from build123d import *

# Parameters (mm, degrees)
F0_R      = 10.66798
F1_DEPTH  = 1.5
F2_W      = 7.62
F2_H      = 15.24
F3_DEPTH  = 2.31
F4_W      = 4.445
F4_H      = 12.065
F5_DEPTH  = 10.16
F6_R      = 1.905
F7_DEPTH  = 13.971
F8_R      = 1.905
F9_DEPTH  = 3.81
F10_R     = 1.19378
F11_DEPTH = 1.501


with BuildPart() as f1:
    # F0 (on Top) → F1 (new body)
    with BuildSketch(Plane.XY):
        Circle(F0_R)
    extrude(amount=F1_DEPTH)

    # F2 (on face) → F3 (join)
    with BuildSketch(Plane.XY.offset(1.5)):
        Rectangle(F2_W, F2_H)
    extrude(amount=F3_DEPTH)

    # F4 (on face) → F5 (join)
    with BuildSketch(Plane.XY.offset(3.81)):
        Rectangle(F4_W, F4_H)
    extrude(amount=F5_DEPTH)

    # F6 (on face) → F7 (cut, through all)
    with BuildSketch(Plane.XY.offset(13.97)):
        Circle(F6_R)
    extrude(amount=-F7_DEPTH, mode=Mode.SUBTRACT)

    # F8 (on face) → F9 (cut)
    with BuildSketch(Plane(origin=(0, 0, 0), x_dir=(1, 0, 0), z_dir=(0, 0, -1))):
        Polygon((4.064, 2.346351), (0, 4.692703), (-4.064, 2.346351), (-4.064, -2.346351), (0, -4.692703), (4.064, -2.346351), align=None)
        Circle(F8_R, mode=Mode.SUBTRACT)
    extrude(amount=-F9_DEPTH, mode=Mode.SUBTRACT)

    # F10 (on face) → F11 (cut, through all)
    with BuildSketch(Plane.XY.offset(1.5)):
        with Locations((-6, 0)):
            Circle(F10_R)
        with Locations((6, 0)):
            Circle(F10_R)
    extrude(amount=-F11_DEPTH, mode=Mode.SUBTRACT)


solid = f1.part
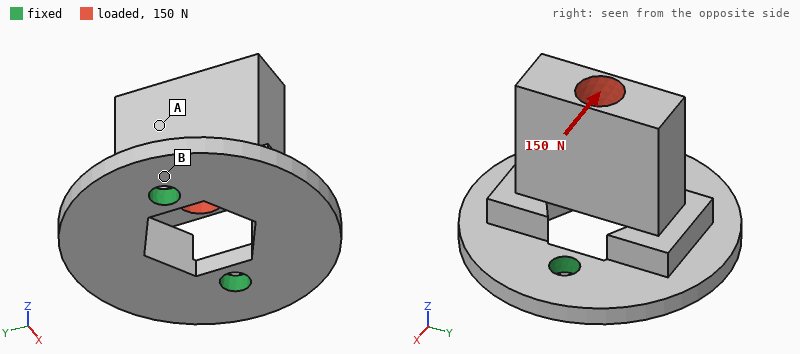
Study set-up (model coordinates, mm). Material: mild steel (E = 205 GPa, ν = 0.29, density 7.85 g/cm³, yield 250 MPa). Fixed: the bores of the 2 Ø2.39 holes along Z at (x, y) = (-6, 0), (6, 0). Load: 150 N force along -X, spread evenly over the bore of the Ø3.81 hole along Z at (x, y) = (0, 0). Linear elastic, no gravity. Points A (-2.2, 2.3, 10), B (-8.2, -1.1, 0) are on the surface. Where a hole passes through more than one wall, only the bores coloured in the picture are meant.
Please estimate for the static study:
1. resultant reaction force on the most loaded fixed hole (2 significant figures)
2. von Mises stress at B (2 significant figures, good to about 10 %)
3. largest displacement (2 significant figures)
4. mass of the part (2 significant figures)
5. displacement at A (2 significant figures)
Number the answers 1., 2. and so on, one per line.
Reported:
1. 130 N
2. 23 MPa
3. 10 µm
4. 7.9 g
5. 6.8 µm
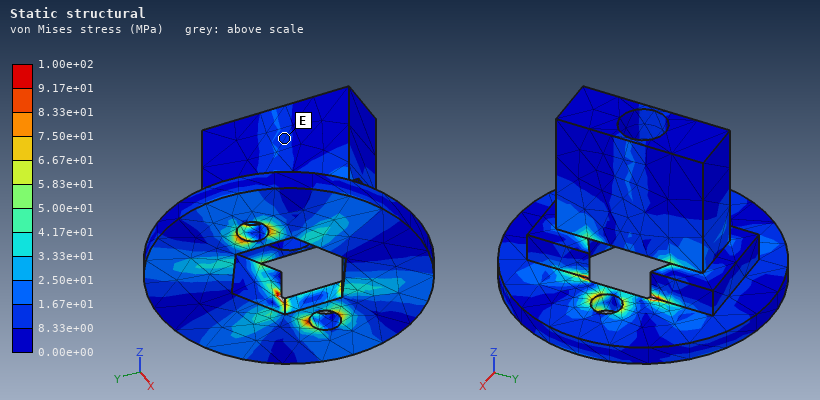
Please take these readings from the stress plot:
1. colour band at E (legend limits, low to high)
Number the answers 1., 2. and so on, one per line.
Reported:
1. 8.33e+00 to 1.67e+01 MPa
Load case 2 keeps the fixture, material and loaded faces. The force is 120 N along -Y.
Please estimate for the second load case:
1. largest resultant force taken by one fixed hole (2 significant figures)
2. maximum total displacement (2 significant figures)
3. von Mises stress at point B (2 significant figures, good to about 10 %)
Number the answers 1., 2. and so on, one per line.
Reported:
1. 60 N
2. 18 µm
3. 29 MPa
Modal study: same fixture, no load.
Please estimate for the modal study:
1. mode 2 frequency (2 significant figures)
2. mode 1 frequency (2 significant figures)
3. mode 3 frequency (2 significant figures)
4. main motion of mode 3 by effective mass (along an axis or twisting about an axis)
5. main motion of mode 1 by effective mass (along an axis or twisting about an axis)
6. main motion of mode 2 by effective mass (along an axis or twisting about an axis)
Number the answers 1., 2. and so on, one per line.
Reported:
1. 12 kHz
2. 6800 Hz
3. 17 kHz
4. along Z
5. along Y
6. along X
